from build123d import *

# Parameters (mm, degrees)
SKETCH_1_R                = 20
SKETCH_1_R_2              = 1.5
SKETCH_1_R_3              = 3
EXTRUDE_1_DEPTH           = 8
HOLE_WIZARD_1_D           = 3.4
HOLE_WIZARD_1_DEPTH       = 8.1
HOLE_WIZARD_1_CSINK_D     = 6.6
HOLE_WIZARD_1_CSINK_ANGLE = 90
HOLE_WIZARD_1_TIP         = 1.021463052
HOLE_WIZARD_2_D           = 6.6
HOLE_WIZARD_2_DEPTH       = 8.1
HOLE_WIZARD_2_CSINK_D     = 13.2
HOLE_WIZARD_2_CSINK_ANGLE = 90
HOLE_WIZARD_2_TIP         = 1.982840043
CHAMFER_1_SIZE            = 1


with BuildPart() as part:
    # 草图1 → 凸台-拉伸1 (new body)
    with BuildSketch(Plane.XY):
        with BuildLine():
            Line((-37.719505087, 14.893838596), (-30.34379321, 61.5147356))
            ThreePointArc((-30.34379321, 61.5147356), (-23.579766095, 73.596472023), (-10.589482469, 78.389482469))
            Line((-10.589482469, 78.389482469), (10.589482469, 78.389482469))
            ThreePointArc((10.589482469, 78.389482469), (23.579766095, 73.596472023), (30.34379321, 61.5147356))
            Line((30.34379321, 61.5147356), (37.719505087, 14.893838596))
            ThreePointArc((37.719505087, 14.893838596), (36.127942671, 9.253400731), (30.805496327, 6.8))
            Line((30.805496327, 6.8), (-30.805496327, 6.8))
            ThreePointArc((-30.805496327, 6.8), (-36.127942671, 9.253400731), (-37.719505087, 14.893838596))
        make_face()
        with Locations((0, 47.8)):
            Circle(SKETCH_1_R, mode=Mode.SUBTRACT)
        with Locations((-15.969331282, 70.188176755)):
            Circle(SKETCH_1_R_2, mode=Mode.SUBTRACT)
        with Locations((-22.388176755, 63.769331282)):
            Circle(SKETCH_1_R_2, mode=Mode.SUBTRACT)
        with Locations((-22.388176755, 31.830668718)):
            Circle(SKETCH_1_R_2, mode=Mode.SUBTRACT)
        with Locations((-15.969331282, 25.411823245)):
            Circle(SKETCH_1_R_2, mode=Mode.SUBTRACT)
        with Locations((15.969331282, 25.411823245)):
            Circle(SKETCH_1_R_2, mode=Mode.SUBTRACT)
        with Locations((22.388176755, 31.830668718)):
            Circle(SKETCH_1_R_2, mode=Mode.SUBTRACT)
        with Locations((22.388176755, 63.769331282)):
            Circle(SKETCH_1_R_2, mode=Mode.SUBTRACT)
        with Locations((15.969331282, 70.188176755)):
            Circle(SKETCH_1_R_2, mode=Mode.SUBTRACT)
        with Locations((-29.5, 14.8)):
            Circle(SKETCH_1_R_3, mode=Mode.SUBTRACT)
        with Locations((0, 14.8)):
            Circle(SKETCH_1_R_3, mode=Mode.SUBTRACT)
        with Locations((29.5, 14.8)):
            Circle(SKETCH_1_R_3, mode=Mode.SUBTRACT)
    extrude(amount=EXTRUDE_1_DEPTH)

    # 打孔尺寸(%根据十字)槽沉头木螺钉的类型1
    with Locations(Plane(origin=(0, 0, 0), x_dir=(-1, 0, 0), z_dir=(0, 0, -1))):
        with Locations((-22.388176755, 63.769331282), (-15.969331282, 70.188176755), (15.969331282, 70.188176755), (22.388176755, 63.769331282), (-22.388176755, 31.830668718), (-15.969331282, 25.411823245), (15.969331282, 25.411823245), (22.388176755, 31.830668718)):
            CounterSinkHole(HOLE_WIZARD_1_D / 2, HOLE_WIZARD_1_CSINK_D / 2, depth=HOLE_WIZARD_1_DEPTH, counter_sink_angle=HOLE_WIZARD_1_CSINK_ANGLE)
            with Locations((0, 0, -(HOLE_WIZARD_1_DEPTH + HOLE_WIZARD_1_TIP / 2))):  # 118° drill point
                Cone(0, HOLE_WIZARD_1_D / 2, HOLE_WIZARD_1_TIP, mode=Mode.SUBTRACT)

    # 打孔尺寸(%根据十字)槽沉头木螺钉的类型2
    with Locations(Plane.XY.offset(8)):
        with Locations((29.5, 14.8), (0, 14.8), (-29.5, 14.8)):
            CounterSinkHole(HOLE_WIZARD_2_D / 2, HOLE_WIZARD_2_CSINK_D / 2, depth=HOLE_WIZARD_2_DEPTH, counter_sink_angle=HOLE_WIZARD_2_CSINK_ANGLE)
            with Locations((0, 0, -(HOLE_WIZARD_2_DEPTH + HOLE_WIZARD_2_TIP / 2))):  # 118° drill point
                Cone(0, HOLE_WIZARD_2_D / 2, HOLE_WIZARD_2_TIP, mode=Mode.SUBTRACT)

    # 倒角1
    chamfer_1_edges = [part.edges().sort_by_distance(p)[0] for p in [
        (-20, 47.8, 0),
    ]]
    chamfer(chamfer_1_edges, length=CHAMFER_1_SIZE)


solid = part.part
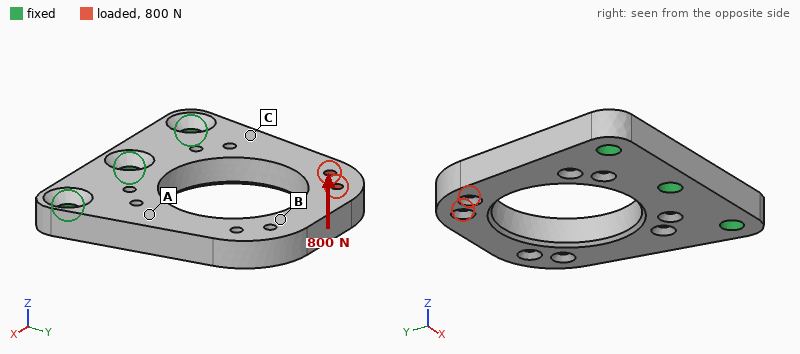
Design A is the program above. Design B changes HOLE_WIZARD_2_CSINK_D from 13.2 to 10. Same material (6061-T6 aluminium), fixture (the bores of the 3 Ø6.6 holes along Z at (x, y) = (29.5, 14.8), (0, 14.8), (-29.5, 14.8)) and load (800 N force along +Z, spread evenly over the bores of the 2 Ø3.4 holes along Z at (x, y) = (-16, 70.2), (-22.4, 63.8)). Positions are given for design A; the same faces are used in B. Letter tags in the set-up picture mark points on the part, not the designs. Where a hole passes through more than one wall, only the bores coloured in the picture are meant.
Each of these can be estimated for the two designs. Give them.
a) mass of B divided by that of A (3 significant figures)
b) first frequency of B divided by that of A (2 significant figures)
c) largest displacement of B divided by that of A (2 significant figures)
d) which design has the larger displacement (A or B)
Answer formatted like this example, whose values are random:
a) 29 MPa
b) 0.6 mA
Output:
a) 1.01
b) 1.1
c) 0.91
d) A
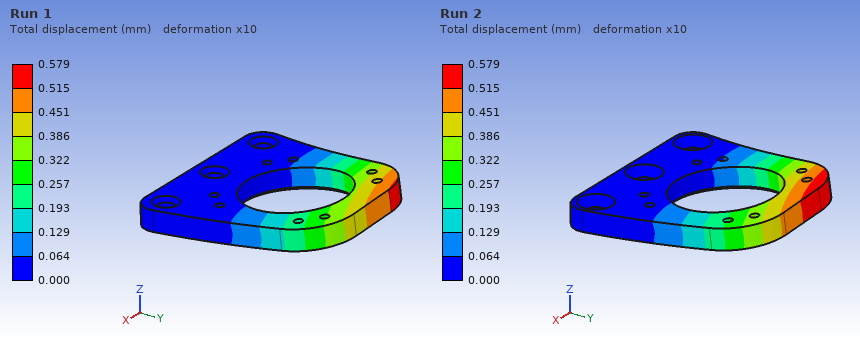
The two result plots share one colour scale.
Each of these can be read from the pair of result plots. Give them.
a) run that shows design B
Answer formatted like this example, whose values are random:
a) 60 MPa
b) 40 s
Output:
a) Run 1
